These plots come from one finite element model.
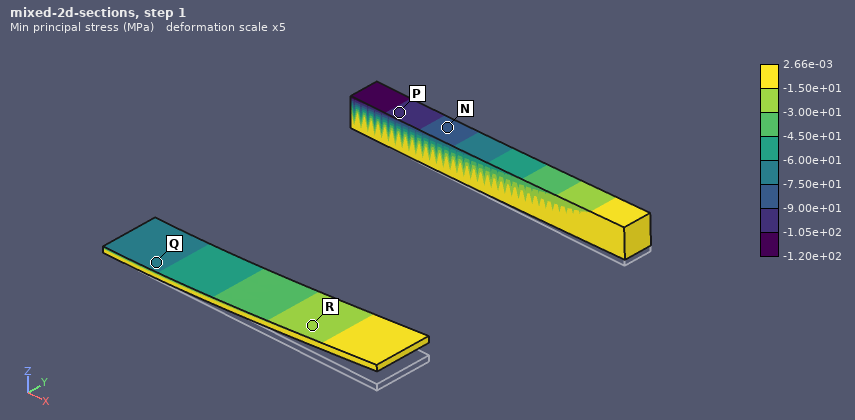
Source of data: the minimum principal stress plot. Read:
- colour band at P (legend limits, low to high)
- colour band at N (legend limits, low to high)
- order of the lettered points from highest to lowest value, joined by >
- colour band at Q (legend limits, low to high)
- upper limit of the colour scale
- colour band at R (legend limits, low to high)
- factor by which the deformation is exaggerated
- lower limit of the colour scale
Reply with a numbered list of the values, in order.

1. -1.05e+02 to -9.00e+01 MPa
2. -9.00e+01 to -7.50e+01 MPa
3. R > Q > N > P
4. -7.50e+01 to -6.00e+01 MPa
5. 2.66e-03 MPa
6. -3.00e+01 to -1.50e+01 MPa
7. 5
8. -1.20e+02 MPa
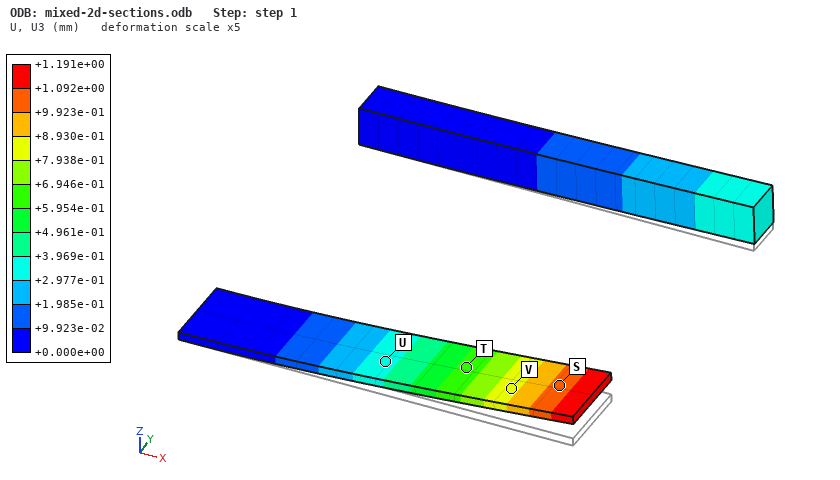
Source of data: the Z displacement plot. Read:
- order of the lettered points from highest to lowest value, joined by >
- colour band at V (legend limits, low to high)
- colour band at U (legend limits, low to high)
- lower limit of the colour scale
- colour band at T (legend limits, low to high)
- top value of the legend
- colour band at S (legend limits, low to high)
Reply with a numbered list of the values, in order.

1. S > V > T > U
2. +7.938e-01 to +8.930e-01 mm
3. +2.977e-01 to +3.969e-01 mm
4. +0.000e+00 mm
5. +5.954e-01 to +6.946e-01 mm
6. +1.191e+00 mm
7. +9.923e-01 to +1.092e+00 mm
